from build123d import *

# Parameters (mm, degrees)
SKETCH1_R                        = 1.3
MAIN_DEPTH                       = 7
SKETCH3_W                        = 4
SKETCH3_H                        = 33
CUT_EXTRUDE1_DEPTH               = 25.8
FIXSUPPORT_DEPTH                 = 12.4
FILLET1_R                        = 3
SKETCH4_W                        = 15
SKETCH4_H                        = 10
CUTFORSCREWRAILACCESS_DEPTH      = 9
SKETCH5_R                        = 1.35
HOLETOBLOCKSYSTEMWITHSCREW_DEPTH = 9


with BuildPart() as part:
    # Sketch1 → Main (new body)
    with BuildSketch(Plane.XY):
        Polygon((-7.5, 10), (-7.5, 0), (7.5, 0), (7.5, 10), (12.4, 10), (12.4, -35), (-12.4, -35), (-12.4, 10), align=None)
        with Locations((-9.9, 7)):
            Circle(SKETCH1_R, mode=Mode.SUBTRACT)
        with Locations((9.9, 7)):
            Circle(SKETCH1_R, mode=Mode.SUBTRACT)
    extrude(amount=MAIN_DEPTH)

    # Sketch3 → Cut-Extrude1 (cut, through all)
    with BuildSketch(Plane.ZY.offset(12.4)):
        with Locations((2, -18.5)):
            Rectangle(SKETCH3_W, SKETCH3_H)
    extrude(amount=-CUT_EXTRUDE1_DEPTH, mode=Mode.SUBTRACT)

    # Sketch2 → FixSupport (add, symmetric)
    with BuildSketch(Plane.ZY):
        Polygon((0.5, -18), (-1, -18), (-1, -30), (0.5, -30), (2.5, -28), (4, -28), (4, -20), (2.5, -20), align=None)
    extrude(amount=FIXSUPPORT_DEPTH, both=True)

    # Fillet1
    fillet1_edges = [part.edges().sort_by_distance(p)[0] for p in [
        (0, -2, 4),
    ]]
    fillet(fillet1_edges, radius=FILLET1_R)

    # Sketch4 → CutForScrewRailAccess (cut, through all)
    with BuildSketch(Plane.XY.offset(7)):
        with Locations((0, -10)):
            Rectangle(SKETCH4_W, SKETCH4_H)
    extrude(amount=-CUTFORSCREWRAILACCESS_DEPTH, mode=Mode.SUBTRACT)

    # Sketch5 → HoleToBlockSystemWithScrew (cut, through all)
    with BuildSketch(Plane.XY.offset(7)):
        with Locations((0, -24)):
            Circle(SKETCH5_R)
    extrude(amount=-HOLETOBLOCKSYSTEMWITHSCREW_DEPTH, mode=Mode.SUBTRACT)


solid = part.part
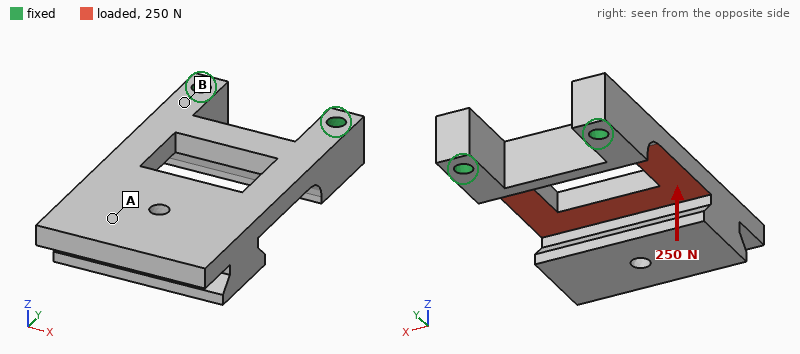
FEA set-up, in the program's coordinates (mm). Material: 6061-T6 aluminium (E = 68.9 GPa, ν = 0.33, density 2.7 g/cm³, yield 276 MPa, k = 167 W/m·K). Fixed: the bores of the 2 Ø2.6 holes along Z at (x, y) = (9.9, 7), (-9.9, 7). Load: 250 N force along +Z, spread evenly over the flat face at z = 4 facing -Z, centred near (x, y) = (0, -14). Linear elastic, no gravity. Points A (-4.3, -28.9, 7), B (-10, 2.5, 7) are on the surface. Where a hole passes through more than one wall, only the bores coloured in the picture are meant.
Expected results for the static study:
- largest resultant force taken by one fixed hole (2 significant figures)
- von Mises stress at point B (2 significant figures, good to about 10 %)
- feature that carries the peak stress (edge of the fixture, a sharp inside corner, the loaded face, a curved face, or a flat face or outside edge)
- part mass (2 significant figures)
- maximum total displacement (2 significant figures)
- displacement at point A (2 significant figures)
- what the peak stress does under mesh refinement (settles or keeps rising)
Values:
130 N
58 MPa
a sharp inside corner
11 g
0.41 mm
0.33 mm
keeps rising
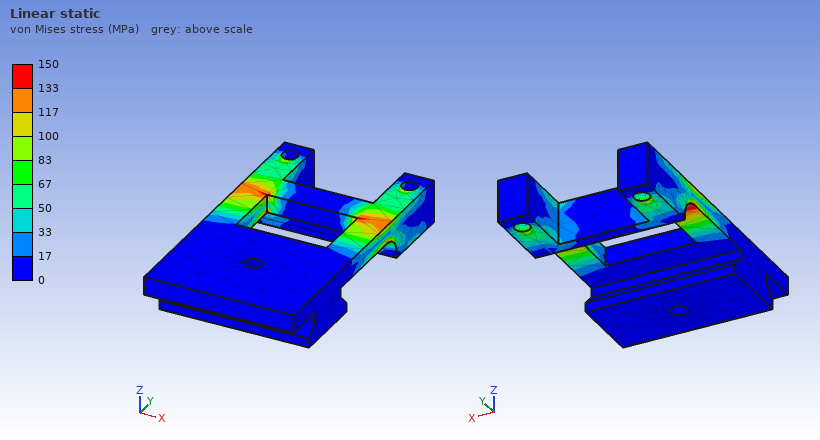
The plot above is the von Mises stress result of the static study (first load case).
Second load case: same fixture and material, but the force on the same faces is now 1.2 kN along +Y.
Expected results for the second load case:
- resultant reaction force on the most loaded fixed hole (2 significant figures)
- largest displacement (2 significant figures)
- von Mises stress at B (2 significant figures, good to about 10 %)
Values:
600 N
0.33 mm
24 MPa
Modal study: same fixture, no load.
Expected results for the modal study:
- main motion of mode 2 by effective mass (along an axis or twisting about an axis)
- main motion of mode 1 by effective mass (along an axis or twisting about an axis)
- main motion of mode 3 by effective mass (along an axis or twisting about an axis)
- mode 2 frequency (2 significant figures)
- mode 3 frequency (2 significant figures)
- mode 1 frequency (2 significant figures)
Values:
along X
along Z
along X
3800 Hz
5200 Hz
1100 Hz
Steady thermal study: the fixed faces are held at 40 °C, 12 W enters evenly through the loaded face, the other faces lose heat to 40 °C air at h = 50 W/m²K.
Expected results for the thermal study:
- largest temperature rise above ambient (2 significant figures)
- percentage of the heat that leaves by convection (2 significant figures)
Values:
29 K
22 %
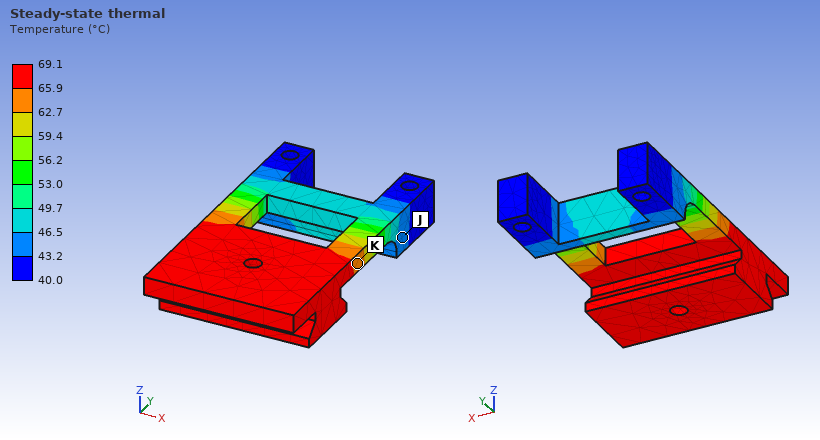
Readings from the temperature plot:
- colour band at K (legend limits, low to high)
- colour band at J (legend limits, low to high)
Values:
62.7 to 65.9 °C
43.2 to 46.5 °C
